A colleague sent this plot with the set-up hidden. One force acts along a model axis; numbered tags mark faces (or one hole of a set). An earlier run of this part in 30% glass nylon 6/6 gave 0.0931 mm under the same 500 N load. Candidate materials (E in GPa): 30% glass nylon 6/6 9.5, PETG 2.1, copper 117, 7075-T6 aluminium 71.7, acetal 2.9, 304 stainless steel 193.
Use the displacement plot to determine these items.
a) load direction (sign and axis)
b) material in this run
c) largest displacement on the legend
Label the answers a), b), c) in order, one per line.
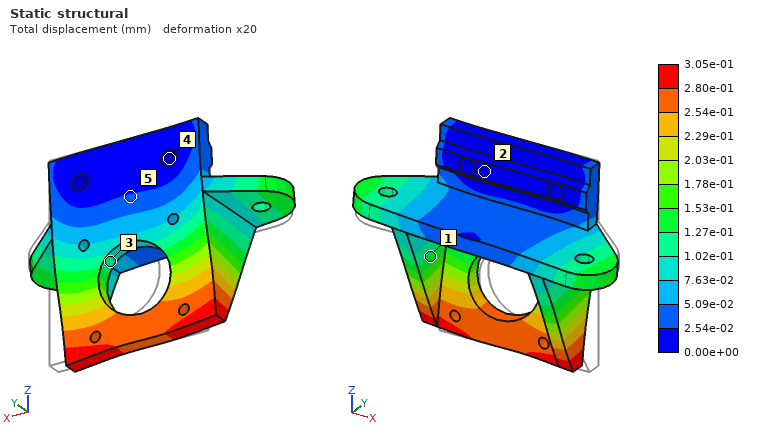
a) -X
b) acetal
c) 3.05e-01 mm
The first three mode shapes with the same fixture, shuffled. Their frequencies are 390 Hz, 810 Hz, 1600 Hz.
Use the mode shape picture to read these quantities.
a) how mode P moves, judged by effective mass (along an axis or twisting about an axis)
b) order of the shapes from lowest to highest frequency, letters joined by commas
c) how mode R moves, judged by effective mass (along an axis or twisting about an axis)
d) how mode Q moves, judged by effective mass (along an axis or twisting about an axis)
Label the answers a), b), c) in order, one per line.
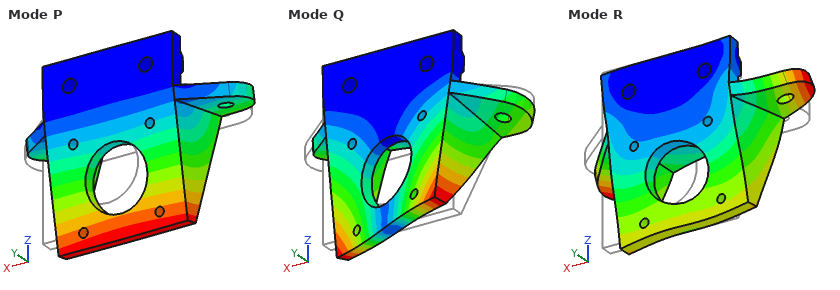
a) along Y
b) P, Q, R
c) along X
d) twisting about Z
